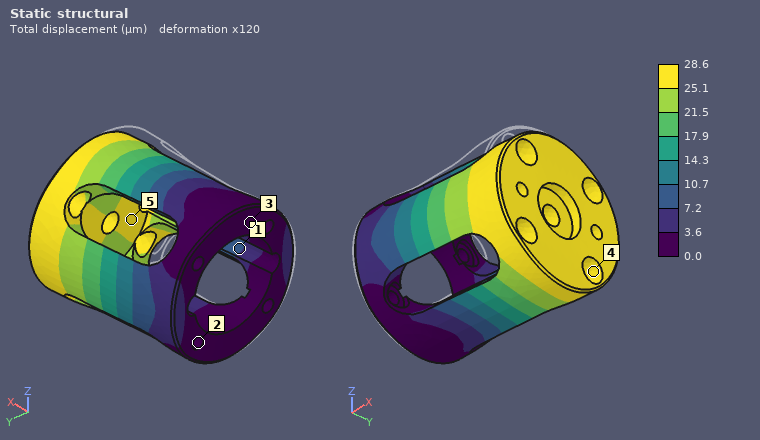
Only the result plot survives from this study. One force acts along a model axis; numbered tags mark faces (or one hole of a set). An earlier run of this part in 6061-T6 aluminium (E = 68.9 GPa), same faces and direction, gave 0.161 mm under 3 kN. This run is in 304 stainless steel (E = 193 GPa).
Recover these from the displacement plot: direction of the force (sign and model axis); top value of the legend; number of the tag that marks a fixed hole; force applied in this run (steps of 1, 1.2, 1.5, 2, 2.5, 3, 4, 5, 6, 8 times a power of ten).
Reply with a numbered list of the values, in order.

1. +Y
2. 28.6 µm
3. 2
4. 1.5 kN
